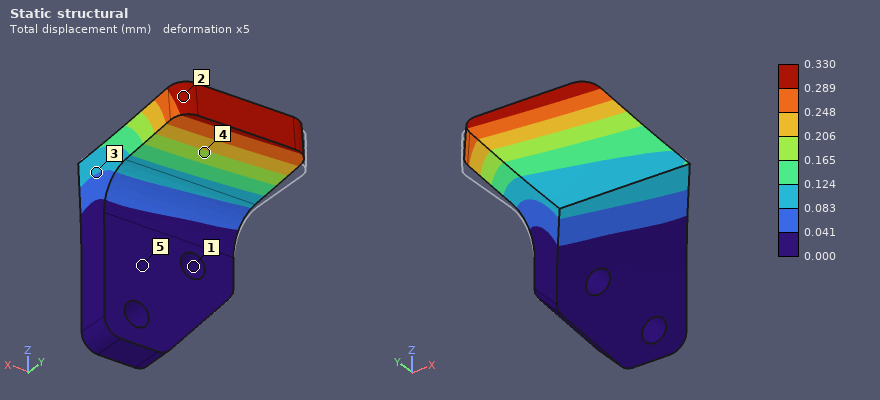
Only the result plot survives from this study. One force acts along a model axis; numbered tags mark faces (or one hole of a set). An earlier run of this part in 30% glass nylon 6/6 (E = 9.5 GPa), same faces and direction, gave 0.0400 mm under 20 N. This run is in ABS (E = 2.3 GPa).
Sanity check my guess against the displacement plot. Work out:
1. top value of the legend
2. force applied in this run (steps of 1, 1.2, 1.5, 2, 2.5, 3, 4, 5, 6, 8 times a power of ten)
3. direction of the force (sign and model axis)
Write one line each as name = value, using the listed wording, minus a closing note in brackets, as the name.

top value of the legend = 0.330 mm
force applied in this run = 40 N
direction of the force = +Z
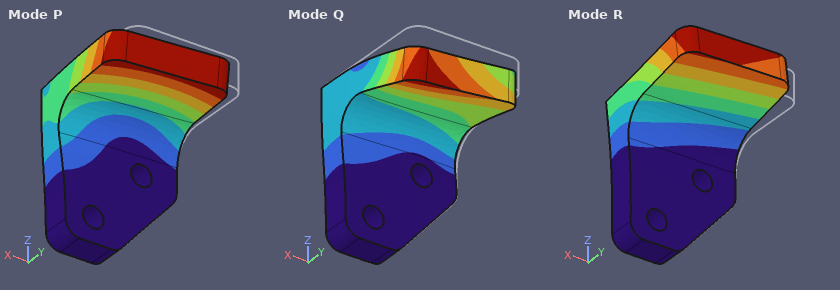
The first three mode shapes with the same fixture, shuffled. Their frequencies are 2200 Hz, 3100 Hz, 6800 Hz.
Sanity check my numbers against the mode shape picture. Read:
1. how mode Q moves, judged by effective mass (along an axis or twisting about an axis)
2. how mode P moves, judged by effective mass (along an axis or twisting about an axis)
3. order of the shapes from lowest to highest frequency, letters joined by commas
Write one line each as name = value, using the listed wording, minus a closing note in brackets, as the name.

how mode Q moves, judged by effective mass = along Y
how mode P moves, judged by effective mass = along X
order of the shapes from lowest to highest frequency, letters joined by commas = R, P, Q
